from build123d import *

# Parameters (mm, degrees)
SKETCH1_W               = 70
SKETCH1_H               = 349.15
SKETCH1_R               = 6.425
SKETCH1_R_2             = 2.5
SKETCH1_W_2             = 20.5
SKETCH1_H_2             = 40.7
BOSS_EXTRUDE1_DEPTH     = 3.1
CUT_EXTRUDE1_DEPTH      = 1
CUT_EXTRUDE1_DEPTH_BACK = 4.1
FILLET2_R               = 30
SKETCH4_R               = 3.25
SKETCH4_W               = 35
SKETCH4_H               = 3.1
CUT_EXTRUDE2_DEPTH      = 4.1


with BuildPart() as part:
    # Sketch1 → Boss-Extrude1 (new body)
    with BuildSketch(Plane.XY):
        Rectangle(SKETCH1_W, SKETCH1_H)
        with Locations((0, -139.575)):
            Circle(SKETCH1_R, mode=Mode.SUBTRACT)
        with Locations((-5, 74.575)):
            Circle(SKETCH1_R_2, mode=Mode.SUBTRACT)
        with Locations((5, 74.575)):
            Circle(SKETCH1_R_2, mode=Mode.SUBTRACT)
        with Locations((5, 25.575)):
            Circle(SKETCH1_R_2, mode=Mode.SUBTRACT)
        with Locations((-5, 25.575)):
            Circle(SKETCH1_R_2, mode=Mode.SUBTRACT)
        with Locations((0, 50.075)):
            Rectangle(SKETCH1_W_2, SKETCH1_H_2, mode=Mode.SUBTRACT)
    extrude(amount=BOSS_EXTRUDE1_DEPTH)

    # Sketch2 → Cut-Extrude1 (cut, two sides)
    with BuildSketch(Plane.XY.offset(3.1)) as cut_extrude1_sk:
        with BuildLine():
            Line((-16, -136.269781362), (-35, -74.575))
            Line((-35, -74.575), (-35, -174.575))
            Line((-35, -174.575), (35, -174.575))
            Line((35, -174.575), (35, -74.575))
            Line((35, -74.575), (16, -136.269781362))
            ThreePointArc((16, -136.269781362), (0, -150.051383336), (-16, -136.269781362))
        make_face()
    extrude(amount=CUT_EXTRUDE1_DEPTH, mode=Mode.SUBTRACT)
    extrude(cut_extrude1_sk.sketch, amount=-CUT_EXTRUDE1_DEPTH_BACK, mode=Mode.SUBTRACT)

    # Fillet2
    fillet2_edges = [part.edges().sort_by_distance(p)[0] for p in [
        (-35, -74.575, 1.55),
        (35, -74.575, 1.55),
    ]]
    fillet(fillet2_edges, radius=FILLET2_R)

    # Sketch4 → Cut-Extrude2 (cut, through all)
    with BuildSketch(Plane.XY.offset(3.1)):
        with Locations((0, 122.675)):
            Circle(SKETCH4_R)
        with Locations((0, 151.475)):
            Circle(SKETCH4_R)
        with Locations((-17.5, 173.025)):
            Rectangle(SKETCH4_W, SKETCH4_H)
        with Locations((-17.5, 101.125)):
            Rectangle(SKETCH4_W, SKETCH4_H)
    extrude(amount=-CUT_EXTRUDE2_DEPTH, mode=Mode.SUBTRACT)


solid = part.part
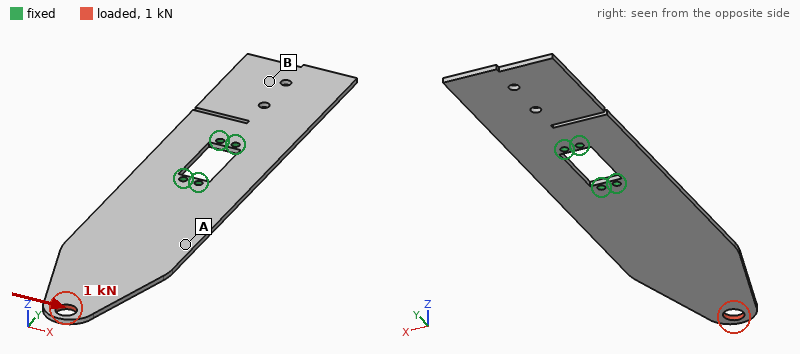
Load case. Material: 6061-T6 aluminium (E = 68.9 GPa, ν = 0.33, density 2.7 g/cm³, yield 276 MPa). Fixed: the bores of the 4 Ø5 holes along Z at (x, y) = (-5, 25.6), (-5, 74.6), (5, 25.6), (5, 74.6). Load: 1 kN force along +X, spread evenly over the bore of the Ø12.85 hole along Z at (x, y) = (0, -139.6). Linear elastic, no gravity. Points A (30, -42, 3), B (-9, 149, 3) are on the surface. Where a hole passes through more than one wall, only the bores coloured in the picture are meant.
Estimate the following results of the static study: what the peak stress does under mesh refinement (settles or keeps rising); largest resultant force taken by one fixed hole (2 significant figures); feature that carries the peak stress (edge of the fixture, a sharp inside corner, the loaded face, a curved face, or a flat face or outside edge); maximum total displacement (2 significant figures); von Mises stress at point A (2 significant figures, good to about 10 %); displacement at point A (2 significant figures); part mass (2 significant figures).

keeps rising
3.5 kN
edge of the fixture
0.60 mm
33 MPa
0.19 mm
160 g
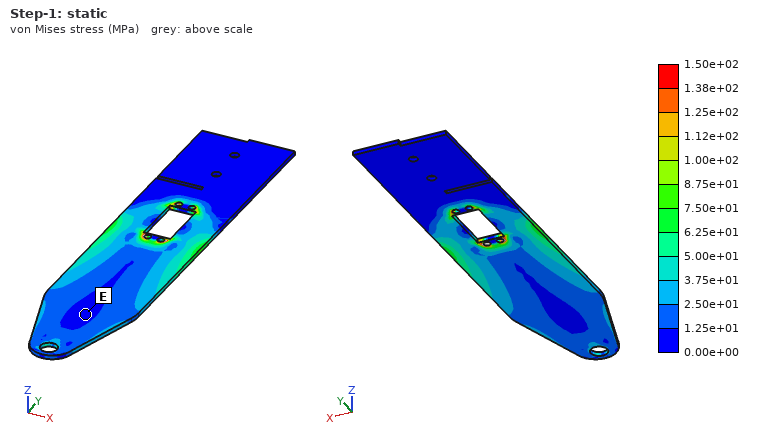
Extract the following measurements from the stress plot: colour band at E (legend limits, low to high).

0.00e+00 to 1.25e+01 MPa
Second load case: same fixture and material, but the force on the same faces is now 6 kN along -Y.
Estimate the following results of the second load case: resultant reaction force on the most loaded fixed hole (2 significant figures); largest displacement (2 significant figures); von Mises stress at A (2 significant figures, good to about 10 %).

2.4 kN
0.12 mm
27 MPa
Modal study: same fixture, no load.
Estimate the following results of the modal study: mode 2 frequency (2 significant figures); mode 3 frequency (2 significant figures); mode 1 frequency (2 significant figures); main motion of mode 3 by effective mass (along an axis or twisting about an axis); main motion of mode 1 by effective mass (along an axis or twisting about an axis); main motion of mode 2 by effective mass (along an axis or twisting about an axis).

210 Hz
530 Hz
110 Hz
twisting about Y
along Z
along Z
